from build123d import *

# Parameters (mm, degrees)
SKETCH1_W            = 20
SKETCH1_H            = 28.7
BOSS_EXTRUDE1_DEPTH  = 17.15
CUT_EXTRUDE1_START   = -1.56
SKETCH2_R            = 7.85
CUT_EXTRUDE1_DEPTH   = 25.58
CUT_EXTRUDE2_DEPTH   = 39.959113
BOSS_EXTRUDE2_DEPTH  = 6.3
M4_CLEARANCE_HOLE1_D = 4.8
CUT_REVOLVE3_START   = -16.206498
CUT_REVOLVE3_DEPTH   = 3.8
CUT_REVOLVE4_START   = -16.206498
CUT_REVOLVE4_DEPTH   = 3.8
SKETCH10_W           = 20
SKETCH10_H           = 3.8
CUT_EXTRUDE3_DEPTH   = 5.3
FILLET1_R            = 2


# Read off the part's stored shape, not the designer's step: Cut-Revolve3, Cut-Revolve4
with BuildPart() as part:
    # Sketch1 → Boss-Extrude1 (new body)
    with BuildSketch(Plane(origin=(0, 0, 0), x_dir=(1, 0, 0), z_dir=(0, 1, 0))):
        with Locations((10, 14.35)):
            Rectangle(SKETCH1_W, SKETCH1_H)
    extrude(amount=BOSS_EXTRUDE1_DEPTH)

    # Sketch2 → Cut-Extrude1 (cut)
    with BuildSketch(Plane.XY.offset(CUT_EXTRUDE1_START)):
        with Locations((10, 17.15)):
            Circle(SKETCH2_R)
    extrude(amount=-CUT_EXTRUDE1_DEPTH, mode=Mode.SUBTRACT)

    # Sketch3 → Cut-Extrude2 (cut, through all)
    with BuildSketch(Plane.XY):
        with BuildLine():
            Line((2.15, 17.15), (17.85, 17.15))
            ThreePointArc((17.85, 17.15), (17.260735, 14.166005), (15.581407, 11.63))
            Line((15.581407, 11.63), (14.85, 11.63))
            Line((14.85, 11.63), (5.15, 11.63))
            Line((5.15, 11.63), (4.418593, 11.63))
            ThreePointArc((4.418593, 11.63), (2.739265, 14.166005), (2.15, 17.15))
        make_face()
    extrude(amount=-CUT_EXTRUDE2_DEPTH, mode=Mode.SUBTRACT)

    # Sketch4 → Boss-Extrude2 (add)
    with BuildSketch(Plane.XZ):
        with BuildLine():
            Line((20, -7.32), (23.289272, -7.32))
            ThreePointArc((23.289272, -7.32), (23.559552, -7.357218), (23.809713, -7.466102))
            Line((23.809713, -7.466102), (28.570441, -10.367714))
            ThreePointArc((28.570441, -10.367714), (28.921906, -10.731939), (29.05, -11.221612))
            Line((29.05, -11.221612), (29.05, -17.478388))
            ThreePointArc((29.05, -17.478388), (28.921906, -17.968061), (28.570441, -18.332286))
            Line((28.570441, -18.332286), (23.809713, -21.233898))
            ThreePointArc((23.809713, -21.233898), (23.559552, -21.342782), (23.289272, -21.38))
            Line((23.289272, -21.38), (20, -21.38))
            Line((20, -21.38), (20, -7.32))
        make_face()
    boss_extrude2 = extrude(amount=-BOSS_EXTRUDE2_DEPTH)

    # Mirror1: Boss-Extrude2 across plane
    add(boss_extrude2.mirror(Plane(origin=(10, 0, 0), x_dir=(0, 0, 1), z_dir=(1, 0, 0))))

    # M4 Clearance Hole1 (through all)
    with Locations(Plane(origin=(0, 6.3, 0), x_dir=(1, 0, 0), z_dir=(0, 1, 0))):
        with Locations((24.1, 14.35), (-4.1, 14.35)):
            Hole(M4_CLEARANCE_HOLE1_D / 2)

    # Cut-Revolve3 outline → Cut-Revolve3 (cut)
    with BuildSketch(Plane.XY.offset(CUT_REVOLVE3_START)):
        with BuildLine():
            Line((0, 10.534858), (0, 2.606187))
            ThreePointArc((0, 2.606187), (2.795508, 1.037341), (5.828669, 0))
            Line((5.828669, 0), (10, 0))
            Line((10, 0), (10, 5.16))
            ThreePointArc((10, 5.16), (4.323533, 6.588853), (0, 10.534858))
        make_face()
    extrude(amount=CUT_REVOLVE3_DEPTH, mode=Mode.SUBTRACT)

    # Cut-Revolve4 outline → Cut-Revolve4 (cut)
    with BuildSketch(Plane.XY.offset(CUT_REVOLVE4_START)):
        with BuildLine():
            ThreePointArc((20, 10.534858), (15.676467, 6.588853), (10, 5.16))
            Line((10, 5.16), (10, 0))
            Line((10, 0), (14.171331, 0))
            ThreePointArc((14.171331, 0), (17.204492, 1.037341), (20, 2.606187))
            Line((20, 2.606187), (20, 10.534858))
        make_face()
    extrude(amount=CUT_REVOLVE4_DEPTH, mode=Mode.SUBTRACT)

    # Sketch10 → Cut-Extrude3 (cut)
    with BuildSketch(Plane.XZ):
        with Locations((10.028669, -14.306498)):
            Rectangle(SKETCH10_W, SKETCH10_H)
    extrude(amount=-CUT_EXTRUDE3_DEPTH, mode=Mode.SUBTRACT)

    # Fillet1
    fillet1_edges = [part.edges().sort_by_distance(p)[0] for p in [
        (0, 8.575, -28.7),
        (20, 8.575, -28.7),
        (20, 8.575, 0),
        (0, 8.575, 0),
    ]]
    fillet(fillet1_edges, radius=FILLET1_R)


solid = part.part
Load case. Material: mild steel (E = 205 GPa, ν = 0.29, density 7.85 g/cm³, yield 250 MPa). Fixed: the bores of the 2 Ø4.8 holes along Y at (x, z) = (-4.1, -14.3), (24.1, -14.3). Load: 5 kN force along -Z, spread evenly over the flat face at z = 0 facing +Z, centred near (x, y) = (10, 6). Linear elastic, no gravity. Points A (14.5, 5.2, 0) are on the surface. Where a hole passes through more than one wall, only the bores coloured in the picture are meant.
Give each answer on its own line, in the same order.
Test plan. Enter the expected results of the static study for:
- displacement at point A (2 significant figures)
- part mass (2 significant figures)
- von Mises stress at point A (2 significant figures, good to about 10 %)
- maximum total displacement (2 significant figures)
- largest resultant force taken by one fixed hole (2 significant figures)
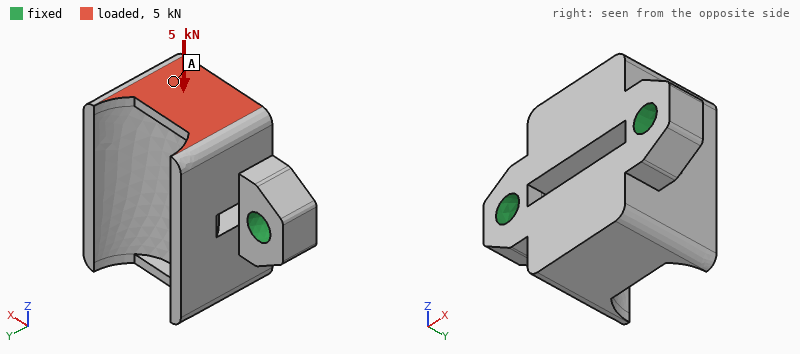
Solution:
11 µm
60 g
26 MPa
17 µm
2.6 kN
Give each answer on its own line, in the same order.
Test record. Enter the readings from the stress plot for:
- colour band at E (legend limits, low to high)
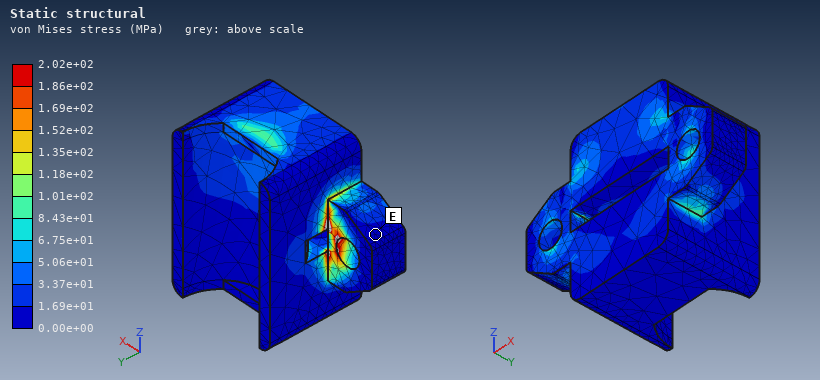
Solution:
0.00e+00 to 1.69e+01 MPa
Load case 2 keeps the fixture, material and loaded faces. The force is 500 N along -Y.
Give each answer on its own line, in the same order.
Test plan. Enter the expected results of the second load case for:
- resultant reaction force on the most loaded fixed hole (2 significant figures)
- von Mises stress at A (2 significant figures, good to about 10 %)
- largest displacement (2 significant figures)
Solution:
300 N
8.8 MPa
6.7 µm
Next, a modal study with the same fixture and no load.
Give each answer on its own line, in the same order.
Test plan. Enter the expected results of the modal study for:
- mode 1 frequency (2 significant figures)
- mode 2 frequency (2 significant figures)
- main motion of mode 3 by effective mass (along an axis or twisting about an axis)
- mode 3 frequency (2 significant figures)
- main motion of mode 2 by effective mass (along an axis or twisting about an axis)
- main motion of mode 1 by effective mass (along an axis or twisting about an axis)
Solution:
11 kHz
21 kHz
along X
28 kHz
along Y
along Z
